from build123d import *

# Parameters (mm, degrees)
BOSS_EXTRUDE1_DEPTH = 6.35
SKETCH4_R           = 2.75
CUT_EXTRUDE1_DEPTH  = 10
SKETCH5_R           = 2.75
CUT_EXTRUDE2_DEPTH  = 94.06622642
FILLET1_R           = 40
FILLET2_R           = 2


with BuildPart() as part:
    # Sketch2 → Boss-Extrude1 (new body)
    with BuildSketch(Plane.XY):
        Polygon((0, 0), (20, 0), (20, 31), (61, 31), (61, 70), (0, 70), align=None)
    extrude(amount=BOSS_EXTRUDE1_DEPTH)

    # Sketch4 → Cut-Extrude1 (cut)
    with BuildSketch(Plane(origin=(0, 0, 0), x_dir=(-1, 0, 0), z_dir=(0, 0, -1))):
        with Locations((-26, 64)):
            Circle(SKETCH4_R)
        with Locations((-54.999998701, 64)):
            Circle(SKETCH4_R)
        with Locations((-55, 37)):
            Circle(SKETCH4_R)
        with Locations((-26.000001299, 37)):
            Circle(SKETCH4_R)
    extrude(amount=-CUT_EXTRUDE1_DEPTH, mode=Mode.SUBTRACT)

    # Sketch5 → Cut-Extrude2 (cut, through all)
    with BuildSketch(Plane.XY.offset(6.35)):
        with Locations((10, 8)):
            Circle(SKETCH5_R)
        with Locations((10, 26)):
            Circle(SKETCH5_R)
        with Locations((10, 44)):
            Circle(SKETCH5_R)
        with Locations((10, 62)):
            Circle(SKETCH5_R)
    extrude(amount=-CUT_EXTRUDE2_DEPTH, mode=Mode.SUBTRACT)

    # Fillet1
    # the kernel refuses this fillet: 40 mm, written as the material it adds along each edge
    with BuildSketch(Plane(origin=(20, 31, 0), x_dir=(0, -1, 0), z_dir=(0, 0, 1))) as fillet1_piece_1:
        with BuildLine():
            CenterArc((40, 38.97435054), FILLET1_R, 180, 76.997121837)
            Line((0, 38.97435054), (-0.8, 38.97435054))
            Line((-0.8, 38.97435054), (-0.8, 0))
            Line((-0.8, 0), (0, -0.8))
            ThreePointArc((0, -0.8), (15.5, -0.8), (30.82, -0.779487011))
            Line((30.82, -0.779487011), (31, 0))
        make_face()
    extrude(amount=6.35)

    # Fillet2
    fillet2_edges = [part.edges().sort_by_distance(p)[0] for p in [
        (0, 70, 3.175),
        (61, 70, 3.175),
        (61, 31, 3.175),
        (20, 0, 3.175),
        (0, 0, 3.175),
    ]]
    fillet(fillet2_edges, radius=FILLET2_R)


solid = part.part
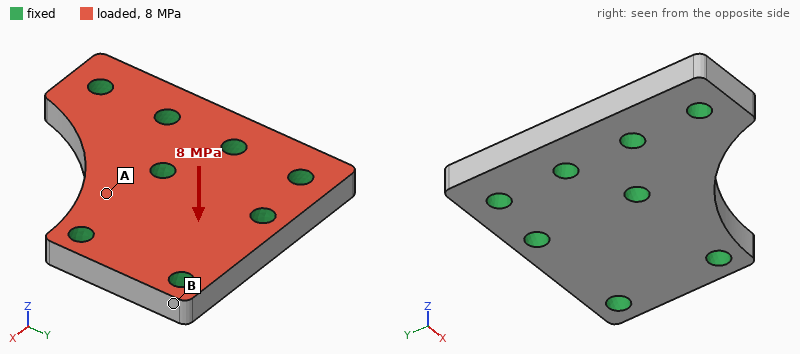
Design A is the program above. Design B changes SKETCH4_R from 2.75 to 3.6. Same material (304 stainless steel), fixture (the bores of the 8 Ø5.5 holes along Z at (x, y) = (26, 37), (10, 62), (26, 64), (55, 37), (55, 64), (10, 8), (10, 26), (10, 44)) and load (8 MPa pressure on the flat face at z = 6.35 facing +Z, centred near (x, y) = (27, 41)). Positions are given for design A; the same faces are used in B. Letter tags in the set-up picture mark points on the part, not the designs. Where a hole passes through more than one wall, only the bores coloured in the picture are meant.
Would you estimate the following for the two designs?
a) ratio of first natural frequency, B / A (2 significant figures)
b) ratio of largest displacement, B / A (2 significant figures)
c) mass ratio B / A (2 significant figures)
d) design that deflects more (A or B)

1.1
0.88
0.98
A
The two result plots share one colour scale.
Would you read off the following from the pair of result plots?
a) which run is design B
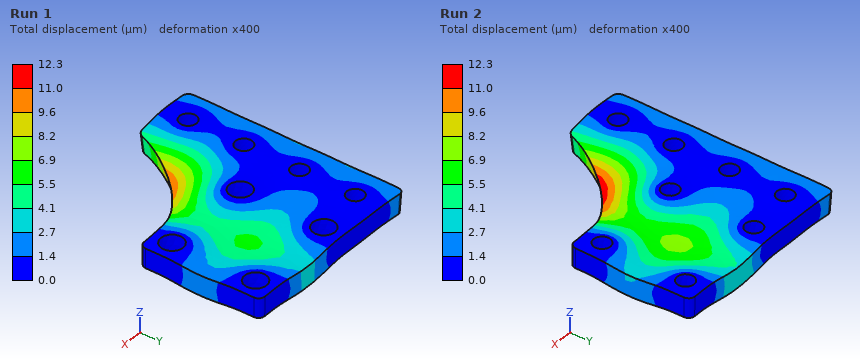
Run 1
